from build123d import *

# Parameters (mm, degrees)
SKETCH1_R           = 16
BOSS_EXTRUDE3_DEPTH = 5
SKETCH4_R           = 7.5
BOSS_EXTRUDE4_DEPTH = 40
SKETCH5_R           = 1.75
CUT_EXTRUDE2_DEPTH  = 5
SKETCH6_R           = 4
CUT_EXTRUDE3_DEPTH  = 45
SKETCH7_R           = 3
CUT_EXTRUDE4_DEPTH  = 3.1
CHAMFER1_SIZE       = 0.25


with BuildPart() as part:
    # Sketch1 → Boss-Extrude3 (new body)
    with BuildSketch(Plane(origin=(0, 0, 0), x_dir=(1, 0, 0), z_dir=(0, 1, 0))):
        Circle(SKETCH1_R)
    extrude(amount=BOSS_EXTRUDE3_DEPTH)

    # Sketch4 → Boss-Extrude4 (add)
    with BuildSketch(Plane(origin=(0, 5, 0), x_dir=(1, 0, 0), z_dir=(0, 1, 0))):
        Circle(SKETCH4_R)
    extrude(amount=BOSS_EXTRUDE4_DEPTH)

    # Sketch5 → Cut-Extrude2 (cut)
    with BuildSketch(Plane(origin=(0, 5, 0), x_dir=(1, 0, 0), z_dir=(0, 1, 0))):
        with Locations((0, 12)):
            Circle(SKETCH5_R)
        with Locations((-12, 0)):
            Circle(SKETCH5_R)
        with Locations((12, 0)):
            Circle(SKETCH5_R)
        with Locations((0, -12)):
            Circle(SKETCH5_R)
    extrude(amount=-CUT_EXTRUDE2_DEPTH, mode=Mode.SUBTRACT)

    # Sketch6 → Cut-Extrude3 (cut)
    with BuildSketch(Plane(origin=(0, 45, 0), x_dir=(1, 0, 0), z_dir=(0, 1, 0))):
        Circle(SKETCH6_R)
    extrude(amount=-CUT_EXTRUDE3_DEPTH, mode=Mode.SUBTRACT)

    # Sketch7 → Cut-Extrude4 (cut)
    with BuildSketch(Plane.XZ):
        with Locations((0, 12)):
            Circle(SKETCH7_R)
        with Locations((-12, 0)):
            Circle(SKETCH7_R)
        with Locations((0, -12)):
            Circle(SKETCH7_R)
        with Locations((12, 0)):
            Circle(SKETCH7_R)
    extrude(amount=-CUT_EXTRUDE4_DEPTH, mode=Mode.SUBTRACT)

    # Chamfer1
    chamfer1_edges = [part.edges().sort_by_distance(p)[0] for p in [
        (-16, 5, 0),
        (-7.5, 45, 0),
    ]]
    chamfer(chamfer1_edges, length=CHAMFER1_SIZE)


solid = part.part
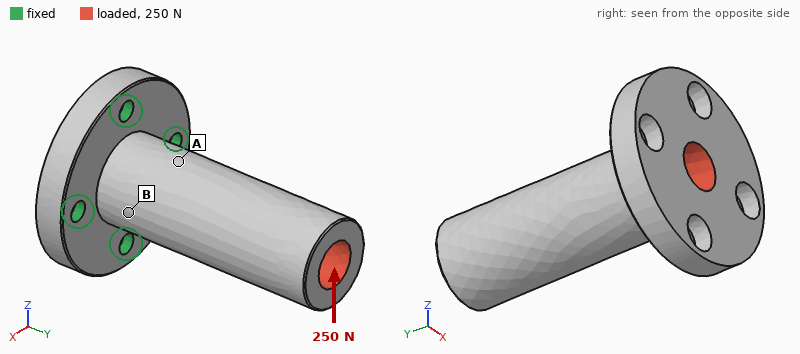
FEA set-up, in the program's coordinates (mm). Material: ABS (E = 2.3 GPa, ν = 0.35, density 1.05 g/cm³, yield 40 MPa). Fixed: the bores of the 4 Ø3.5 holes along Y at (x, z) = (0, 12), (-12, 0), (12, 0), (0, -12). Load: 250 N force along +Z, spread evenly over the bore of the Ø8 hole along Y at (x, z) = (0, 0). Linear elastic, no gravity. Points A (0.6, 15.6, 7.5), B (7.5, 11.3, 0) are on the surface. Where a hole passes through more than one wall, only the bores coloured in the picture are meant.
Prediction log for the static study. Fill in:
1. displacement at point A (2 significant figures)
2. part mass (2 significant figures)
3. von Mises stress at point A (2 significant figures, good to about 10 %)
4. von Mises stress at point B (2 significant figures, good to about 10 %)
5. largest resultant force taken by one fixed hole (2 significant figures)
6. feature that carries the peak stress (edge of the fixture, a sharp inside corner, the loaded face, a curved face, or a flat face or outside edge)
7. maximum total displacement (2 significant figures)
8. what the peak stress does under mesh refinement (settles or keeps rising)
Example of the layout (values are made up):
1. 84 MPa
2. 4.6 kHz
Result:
1. 0.21 mm
2. 8.8 g
3. 7.6 MPa
4. 3.1 MPa
5. 200 N
6. edge of the fixture
7. 0.77 mm
8. keeps rising
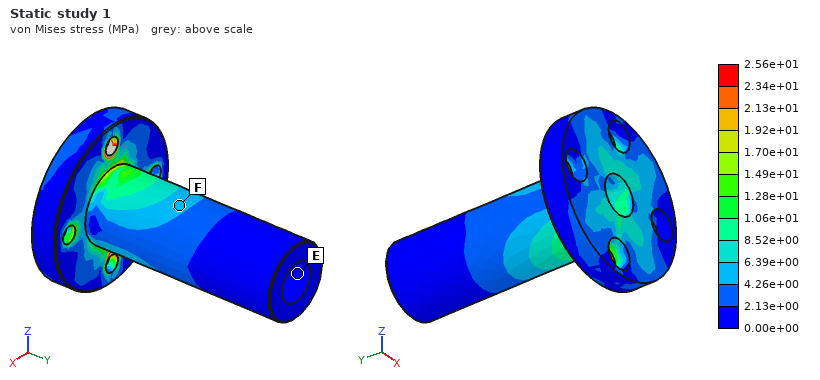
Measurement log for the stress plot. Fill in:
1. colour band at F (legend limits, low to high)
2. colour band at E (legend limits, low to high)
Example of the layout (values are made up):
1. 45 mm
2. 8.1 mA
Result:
1. 4.26e+00 to 6.39e+00 MPa
2. 0.00e+00 to 2.13e+00 MPa
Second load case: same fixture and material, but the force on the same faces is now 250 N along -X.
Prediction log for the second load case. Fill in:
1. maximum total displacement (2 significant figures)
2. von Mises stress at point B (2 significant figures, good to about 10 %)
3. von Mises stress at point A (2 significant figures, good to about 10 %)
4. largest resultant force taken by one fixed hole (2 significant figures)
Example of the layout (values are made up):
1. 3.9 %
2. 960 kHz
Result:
1. 0.76 mm
2. 9.8 MPa
3. 3.5 MPa
4. 200 N
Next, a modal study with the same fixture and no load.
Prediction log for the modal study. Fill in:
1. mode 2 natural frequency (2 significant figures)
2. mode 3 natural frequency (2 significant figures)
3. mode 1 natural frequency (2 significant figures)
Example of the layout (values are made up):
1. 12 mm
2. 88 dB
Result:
1. 1400 Hz
2. 5300 Hz
3. 1400 Hz
